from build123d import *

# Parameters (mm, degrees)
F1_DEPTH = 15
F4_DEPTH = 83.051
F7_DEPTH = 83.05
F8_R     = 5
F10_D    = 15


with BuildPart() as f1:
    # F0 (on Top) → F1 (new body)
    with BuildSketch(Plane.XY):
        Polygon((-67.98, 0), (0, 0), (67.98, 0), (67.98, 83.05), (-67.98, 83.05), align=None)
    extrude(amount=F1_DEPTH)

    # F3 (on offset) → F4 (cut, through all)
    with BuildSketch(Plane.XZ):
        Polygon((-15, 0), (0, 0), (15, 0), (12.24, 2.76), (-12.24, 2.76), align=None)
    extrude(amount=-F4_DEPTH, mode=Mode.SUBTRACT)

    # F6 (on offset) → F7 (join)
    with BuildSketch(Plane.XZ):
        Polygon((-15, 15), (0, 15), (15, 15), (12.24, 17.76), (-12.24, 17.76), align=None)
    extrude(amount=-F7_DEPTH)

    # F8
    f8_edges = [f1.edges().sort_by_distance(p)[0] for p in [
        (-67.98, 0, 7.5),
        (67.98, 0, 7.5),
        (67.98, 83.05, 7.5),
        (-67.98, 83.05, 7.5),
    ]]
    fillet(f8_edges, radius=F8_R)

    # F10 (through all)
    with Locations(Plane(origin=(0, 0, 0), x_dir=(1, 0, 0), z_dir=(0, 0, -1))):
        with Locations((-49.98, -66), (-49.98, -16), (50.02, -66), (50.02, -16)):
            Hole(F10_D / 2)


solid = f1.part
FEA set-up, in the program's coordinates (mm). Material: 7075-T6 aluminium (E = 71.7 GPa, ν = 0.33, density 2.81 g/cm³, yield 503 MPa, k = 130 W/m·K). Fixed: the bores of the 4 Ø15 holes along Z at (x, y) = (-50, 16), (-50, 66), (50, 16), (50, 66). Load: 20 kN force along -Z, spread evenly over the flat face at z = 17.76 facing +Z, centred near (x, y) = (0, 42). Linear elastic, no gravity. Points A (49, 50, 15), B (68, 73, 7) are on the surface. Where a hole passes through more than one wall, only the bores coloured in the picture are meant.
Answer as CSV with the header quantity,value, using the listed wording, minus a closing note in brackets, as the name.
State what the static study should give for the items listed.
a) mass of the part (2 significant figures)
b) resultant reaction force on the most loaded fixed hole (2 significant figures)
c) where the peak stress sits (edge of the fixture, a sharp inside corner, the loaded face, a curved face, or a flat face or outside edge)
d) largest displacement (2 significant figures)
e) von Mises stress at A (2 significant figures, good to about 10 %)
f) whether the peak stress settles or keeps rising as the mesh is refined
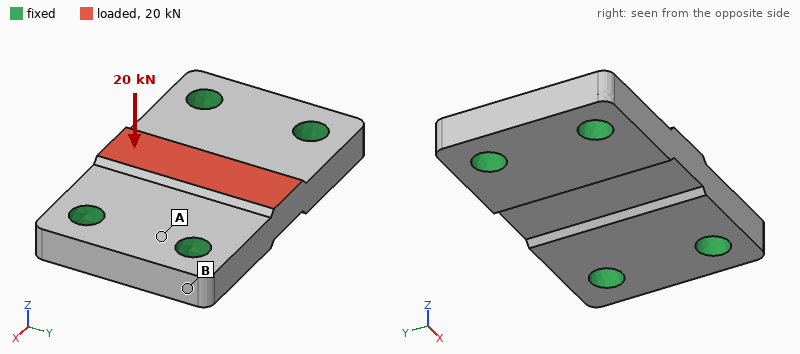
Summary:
quantity,value
mass of the part,450 g
resultant reaction force on the most loaded fixed hole,5.9 kN
where the peak stress sits,edge of the fixture
largest displacement,63 µm
von Mises stress at A,20 MPa
whether the peak stress settles or keeps rising as the mesh is refined,keeps rising
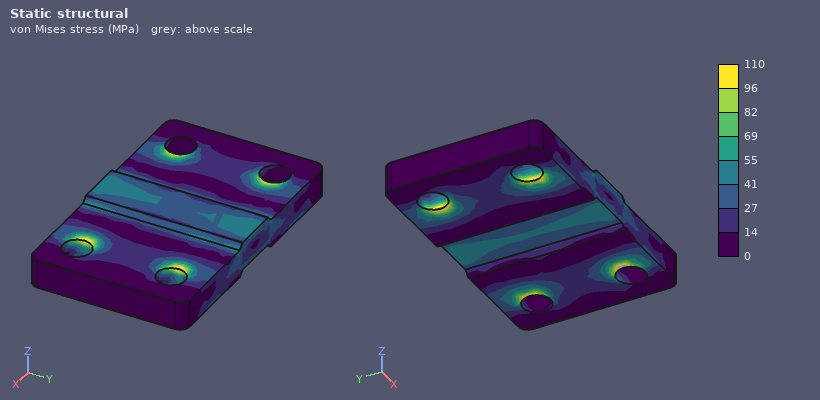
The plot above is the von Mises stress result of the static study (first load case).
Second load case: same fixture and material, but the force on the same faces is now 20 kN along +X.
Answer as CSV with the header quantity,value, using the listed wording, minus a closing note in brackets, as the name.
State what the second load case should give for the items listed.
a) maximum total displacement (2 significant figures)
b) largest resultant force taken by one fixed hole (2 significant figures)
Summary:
quantity,value
maximum total displacement,9.8 µm
largest resultant force taken by one fixed hole,5.3 kN
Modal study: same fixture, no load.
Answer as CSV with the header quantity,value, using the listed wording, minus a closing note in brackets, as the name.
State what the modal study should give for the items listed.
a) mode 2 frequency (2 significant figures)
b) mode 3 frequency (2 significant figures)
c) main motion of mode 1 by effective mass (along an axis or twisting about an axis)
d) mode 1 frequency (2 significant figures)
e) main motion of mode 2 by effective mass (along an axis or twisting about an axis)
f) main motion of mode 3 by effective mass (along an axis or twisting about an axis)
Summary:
quantity,value
mode 2 frequency,9400 Hz
mode 3 frequency,15 kHz
main motion of mode 1 by effective mass,along Z
mode 1 frequency,7700 Hz
main motion of mode 2 by effective mass,twisting about X
main motion of mode 3 by effective mass,along Y
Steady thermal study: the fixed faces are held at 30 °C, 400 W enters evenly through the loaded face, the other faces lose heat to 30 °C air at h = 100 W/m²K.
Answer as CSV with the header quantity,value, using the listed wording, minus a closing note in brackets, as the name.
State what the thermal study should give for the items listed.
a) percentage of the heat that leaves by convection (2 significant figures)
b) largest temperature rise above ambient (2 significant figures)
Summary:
quantity,value
percentage of the heat that leaves by convection,11 %
largest temperature rise above ambient,57 K
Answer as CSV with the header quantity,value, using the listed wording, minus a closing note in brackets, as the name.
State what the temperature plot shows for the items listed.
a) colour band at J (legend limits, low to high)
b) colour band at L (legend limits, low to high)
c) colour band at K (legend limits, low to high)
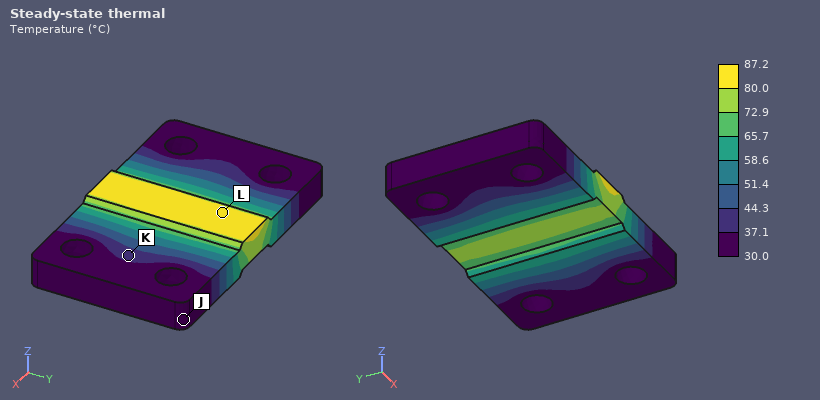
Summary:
quantity,value
colour band at J,30.0 to 37.1 °C
colour band at L,80.0 to 87.2 °C
colour band at K,37.1 to 44.3 °C
